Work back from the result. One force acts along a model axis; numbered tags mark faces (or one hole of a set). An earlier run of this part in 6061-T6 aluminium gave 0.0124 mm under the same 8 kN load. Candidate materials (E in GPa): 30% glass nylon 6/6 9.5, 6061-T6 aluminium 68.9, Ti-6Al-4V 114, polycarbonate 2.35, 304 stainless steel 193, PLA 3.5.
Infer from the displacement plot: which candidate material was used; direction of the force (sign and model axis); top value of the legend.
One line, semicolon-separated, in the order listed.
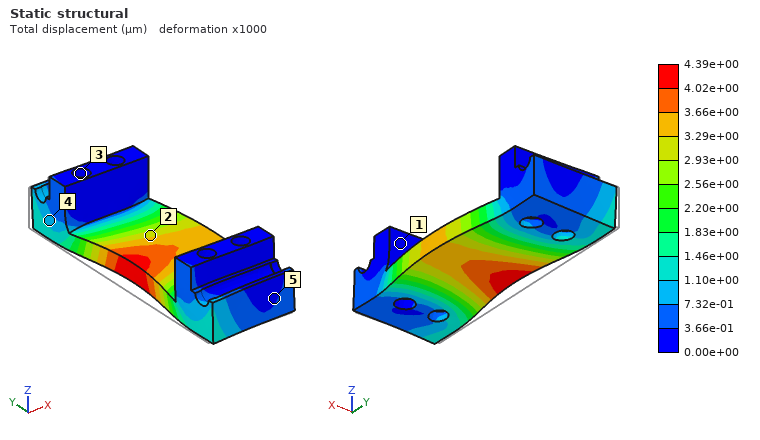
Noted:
304 stainless steel; +X; 4.39e+00 µm
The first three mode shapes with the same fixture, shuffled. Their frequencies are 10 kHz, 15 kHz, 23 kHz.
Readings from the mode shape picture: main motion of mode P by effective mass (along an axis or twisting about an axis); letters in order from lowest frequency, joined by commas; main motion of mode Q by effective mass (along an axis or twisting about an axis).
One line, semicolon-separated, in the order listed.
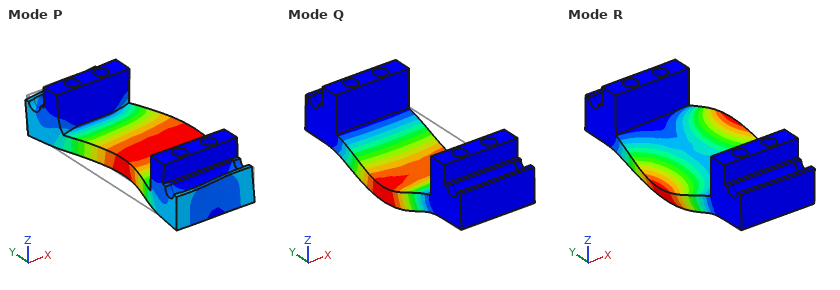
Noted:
along X; Q, R, P; along Z
